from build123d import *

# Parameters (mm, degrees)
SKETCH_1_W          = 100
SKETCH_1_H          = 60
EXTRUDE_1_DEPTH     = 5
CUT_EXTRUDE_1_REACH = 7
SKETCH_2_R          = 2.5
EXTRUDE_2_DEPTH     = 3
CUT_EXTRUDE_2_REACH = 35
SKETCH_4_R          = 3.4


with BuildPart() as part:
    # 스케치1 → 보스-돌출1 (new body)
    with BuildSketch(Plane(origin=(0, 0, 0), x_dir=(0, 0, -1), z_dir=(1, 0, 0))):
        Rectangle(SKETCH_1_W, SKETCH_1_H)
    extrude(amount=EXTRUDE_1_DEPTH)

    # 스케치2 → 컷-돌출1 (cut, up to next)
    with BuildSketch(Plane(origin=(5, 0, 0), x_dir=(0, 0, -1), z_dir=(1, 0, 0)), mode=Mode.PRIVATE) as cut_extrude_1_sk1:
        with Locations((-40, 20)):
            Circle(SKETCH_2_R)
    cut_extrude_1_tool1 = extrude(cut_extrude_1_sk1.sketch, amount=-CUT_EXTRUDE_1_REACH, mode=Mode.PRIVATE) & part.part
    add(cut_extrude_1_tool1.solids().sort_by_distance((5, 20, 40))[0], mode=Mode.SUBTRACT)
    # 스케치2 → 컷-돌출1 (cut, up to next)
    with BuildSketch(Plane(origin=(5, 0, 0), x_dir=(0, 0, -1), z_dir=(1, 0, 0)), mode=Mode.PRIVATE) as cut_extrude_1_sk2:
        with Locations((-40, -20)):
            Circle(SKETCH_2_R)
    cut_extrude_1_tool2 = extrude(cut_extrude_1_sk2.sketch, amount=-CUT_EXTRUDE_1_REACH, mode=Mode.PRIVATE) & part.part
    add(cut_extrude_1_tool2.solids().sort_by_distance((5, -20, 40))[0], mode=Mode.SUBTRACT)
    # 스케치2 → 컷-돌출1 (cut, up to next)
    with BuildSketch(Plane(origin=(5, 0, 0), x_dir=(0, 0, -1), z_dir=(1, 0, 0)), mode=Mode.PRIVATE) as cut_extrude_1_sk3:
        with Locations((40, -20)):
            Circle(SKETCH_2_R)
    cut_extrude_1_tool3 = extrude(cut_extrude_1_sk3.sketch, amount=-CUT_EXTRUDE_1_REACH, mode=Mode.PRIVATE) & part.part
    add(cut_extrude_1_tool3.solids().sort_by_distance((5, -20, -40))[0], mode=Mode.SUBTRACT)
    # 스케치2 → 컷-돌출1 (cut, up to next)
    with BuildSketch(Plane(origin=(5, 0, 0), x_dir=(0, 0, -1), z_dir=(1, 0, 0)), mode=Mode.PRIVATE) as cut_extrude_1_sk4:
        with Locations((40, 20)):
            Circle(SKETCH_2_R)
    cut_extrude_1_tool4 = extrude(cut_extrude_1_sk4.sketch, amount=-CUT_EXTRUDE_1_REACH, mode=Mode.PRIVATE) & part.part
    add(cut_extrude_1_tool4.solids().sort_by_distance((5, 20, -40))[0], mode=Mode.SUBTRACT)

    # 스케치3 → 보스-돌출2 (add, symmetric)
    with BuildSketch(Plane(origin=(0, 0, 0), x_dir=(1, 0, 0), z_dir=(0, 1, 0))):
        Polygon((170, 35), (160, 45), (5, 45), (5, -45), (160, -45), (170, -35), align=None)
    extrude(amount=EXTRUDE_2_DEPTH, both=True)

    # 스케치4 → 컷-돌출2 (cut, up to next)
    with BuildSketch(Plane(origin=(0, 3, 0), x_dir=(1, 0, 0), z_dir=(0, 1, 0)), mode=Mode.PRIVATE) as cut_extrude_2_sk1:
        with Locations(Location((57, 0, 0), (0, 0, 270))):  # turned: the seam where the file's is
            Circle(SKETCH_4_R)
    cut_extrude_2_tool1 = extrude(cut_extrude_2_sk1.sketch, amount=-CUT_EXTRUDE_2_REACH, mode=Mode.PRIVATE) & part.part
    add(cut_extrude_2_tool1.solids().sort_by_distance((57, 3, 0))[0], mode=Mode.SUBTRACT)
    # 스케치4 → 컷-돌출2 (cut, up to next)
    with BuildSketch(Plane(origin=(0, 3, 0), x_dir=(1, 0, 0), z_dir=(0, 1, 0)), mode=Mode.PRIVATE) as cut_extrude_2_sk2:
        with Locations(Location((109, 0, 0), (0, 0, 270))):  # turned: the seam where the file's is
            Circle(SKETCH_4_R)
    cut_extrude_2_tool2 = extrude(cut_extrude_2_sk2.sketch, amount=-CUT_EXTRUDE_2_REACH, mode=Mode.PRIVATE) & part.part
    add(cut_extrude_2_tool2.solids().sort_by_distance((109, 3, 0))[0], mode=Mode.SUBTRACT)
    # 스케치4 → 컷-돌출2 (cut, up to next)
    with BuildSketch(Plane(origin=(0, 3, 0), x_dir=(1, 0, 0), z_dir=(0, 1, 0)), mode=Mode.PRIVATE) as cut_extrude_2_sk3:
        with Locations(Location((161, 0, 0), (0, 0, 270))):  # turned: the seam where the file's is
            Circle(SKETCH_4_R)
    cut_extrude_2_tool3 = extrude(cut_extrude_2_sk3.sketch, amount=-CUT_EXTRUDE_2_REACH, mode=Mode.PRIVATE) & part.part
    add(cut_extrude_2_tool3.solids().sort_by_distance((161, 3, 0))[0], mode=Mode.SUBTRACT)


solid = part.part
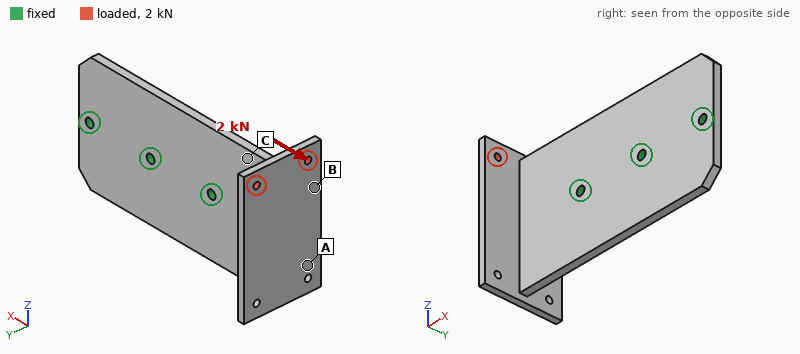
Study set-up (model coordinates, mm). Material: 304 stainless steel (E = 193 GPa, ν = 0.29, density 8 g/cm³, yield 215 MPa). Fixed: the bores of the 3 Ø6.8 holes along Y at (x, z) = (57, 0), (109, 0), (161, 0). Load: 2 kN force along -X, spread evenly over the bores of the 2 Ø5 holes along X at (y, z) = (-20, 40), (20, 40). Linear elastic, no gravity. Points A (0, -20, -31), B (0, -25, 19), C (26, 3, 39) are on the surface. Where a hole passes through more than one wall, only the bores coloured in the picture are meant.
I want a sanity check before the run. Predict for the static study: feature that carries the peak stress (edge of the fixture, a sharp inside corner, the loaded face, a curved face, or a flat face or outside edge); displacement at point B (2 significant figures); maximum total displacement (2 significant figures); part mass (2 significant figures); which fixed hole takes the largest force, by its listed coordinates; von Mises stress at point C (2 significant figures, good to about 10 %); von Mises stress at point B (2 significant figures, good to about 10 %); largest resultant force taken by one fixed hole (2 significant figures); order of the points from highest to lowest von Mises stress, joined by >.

a flat face or outside edge
25 µm
71 µm
940 g
(57, 0)
15 MPa
34 MPa
1.6 kN
B > C > A
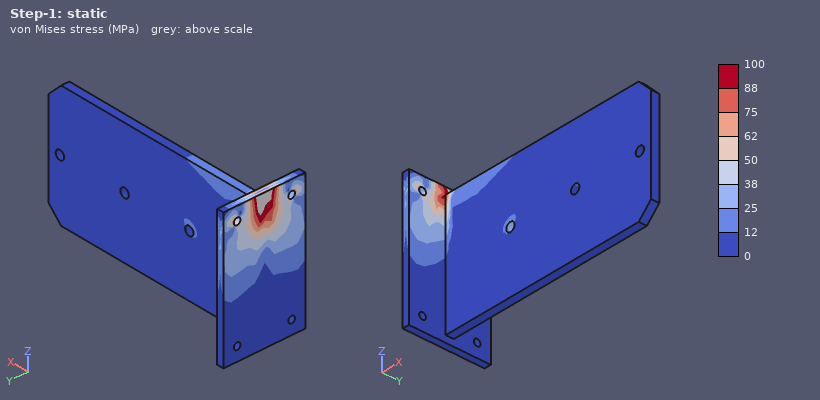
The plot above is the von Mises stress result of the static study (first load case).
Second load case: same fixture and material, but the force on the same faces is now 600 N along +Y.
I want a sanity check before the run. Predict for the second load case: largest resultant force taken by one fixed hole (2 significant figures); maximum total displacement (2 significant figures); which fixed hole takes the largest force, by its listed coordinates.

900 N
0.31 mm
(57, 0)
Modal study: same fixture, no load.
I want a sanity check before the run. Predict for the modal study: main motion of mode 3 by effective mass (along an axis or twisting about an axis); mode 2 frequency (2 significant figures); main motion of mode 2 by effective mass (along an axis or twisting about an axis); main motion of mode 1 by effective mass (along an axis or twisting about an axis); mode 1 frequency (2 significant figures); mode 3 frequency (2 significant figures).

twisting about X
810 Hz
twisting about X
along Y
590 Hz
2100 Hz
